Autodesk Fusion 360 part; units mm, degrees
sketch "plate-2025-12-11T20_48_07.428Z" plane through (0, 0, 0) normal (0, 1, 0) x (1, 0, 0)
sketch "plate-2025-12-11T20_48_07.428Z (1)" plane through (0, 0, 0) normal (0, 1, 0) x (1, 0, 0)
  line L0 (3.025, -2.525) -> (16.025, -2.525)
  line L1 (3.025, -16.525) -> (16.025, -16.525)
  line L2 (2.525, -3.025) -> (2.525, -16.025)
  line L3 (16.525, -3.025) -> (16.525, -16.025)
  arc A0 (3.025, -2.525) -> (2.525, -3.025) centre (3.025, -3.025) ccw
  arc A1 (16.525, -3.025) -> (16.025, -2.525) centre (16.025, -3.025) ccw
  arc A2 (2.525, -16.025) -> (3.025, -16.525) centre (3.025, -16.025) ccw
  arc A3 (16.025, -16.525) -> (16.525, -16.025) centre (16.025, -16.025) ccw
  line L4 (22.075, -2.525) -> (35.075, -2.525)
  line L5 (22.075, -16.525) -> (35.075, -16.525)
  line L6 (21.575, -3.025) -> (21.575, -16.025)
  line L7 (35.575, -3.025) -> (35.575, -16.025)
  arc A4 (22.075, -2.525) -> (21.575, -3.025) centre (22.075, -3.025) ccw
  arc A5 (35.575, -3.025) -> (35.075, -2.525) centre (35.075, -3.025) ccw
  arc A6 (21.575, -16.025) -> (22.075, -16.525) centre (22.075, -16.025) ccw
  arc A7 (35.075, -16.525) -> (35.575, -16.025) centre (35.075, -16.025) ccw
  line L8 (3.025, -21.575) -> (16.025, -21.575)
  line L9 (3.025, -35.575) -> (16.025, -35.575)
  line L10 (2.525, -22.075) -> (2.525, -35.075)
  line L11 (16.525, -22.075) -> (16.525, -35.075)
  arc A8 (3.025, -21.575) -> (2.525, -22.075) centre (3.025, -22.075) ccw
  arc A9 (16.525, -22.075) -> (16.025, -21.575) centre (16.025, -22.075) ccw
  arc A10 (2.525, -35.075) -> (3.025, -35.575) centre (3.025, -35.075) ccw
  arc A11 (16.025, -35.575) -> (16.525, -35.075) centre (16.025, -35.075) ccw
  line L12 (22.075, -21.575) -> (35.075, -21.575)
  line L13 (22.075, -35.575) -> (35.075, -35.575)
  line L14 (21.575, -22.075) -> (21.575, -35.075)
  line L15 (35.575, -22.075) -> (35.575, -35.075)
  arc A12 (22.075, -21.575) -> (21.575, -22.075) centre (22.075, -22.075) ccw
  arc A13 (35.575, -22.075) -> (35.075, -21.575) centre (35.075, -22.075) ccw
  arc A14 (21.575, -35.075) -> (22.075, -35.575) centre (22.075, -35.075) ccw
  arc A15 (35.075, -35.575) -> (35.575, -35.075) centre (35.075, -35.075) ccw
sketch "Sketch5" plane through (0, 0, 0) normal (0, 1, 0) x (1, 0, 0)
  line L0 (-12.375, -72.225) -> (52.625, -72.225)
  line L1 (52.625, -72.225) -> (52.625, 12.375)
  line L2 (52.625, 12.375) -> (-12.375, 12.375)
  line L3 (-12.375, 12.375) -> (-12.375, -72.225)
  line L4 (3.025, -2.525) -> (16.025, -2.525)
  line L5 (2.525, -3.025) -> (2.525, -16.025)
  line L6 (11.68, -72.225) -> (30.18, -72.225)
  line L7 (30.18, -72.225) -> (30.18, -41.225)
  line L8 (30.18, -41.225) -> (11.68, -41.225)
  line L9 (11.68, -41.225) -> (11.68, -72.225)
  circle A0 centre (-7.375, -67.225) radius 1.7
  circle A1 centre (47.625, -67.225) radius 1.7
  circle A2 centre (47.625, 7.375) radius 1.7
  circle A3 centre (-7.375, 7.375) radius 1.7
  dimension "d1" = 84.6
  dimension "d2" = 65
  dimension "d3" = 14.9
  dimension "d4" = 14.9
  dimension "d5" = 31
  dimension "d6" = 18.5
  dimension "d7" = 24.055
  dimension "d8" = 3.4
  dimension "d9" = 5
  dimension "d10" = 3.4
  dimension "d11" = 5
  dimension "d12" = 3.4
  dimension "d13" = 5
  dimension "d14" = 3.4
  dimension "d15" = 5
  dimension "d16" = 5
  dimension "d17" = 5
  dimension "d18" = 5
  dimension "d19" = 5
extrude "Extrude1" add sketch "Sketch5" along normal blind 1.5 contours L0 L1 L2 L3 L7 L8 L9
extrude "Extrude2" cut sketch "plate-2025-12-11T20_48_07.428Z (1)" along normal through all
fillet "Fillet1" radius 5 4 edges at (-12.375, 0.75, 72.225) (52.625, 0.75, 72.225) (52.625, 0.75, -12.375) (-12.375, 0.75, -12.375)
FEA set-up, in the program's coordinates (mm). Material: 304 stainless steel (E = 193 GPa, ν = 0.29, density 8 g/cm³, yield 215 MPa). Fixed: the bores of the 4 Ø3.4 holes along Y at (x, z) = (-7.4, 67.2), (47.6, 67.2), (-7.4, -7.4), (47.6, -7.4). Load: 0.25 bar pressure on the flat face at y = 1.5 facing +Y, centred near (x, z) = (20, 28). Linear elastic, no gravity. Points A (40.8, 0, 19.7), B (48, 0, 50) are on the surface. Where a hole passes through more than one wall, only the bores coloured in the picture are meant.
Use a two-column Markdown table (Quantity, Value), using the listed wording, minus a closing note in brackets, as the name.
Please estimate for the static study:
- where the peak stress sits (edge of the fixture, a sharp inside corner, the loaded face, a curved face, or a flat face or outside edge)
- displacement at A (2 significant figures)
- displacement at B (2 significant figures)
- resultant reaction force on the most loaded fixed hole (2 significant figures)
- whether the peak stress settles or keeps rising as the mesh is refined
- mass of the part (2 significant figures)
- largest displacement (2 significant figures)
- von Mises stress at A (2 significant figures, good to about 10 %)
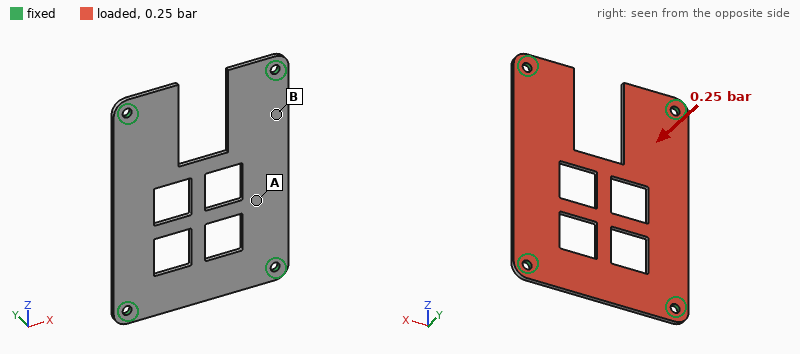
| Quantity | Value |
|---|---|
| where the peak stress sits | edge of the fixture |
| displacement at A | 43 µm |
| displacement at B | 22 µm |
| resultant reaction force on the most loaded fixed hole | 27 N |
| whether the peak stress settles or keeps rising as the mesh is refined | keeps rising |
| mass of the part | 49 g |
| largest displacement | 63 µm |
| von Mises stress at A | 14 MPa |
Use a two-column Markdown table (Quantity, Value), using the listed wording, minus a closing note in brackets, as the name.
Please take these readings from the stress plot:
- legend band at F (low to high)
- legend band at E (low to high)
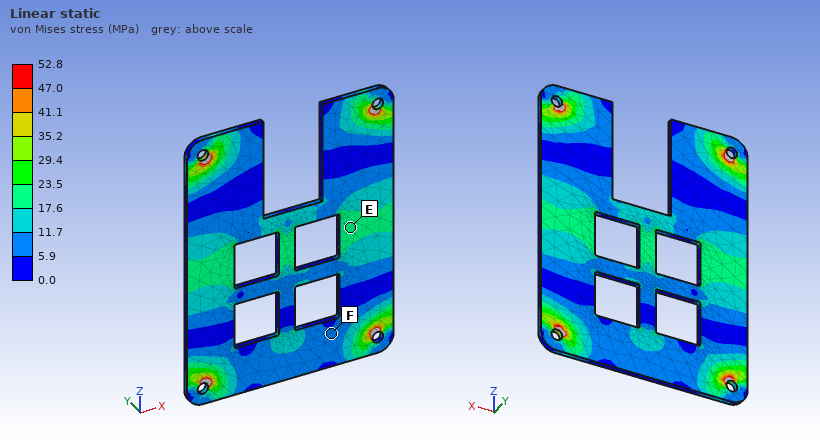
| Quantity | Value |
|---|---|
| legend band at F | 5.9 to 11.7 MPa |
| legend band at E | 17.6 to 23.5 MPa |
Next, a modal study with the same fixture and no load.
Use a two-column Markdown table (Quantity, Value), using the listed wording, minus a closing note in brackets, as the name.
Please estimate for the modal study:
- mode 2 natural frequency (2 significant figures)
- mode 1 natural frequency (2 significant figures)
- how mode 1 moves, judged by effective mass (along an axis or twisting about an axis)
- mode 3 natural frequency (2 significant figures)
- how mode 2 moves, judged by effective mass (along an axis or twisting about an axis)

| Quantity | Value |
|---|---|
| mode 2 natural frequency | 1600 Hz |
| mode 1 natural frequency | 1200 Hz |
| how mode 1 moves, judged by effective mass | along Y |
| mode 3 natural frequency | 2300 Hz |
| how mode 2 moves, judged by effective mass | twisting about Z |
